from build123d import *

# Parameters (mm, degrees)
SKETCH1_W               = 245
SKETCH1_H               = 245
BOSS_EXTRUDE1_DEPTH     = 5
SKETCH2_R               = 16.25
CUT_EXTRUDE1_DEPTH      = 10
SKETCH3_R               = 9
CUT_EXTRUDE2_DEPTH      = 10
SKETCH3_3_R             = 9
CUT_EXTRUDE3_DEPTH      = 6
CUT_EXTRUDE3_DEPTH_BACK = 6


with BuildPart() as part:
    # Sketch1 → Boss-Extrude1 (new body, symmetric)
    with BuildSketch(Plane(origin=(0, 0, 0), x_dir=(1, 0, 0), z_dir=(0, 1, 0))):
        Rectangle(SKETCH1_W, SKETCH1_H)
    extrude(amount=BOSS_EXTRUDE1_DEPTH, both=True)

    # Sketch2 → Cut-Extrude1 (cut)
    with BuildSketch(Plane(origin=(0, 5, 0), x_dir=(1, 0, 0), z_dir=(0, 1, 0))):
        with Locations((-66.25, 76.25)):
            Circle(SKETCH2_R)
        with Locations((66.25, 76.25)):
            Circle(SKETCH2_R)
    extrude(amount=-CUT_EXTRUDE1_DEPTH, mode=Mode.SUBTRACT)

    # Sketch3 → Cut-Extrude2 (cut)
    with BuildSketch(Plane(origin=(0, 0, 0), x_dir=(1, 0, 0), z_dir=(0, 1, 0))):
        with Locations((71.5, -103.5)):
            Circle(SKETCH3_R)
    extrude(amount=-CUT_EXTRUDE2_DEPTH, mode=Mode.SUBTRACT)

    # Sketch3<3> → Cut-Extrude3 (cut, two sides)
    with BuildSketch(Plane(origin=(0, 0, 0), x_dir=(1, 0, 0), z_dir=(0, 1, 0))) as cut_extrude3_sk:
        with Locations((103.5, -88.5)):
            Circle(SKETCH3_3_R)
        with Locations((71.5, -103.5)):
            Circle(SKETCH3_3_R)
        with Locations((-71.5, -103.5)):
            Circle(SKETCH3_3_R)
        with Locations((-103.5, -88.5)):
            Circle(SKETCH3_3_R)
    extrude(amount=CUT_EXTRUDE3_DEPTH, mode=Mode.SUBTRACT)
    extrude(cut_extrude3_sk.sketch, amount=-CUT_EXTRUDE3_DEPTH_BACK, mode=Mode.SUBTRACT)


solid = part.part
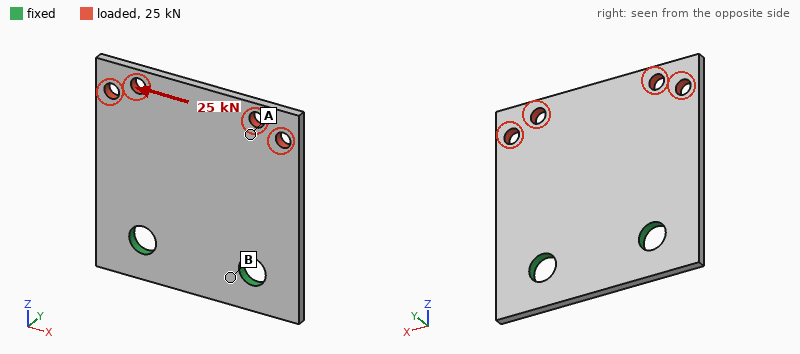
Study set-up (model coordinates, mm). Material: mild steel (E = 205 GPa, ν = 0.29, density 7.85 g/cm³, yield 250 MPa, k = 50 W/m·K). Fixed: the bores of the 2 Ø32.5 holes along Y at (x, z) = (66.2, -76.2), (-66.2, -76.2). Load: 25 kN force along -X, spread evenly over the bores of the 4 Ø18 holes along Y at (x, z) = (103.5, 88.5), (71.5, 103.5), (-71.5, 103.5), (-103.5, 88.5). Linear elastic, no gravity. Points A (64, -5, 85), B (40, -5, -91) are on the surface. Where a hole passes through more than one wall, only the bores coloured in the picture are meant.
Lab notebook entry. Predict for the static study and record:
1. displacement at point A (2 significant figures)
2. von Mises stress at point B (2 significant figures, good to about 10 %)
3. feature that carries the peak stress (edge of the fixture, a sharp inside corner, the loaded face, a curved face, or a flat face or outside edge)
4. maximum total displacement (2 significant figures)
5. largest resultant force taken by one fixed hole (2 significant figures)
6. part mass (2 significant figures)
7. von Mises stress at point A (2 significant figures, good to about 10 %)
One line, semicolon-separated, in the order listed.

48 µm; 8.8 MPa; edge of the fixture; 65 µm; 30 kN; 4.5 kg; 26 MPa
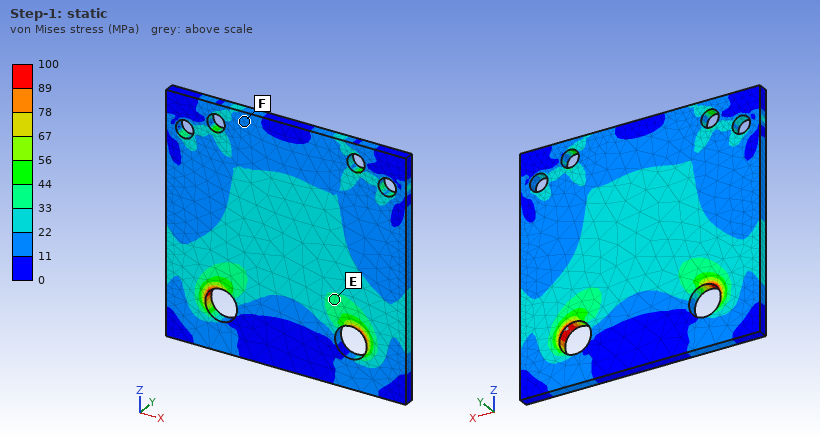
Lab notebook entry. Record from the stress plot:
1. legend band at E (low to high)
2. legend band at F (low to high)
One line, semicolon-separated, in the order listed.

33 to 44 MPa; 11 to 22 MPa
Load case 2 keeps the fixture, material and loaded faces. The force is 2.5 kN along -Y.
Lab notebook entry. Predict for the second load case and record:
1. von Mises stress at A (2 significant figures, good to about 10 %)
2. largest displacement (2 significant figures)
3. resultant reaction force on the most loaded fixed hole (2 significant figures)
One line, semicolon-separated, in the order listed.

11 MPa; 1.1 mm; 1.3 kN
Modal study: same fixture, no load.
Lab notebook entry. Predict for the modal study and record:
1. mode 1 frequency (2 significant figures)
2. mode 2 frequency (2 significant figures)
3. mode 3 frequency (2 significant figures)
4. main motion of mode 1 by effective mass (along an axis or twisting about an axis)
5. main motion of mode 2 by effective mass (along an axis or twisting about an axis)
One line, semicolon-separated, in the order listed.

240 Hz; 480 Hz; 1100 Hz; along Y; twisting about Z
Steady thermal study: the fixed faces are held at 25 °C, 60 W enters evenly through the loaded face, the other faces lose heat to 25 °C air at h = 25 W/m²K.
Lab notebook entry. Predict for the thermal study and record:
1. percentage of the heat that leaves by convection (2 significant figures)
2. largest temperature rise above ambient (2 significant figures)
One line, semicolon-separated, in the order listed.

74 %; 48 K
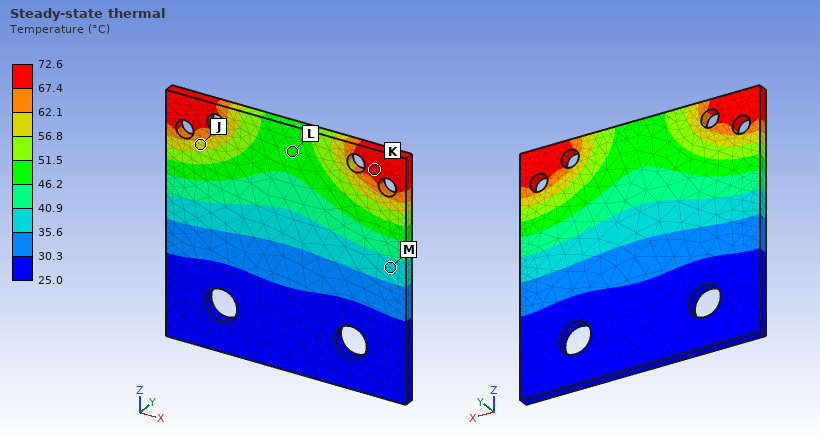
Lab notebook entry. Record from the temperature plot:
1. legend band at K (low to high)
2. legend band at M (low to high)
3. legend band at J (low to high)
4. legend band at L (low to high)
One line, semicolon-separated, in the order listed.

67.4 to 72.6 °C; 35.6 to 40.9 °C; 56.8 to 62.1 °C; 46.2 to 51.5 °C
